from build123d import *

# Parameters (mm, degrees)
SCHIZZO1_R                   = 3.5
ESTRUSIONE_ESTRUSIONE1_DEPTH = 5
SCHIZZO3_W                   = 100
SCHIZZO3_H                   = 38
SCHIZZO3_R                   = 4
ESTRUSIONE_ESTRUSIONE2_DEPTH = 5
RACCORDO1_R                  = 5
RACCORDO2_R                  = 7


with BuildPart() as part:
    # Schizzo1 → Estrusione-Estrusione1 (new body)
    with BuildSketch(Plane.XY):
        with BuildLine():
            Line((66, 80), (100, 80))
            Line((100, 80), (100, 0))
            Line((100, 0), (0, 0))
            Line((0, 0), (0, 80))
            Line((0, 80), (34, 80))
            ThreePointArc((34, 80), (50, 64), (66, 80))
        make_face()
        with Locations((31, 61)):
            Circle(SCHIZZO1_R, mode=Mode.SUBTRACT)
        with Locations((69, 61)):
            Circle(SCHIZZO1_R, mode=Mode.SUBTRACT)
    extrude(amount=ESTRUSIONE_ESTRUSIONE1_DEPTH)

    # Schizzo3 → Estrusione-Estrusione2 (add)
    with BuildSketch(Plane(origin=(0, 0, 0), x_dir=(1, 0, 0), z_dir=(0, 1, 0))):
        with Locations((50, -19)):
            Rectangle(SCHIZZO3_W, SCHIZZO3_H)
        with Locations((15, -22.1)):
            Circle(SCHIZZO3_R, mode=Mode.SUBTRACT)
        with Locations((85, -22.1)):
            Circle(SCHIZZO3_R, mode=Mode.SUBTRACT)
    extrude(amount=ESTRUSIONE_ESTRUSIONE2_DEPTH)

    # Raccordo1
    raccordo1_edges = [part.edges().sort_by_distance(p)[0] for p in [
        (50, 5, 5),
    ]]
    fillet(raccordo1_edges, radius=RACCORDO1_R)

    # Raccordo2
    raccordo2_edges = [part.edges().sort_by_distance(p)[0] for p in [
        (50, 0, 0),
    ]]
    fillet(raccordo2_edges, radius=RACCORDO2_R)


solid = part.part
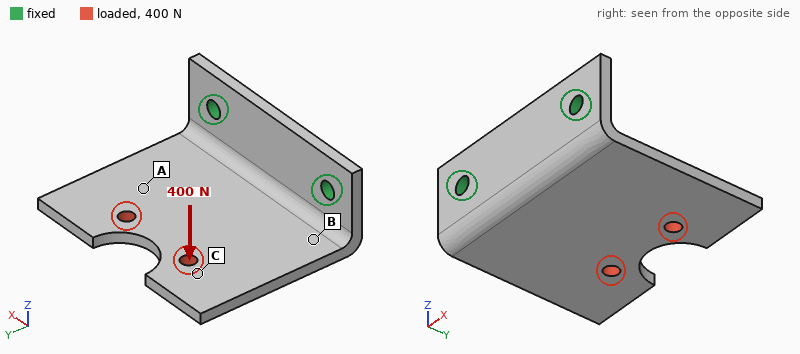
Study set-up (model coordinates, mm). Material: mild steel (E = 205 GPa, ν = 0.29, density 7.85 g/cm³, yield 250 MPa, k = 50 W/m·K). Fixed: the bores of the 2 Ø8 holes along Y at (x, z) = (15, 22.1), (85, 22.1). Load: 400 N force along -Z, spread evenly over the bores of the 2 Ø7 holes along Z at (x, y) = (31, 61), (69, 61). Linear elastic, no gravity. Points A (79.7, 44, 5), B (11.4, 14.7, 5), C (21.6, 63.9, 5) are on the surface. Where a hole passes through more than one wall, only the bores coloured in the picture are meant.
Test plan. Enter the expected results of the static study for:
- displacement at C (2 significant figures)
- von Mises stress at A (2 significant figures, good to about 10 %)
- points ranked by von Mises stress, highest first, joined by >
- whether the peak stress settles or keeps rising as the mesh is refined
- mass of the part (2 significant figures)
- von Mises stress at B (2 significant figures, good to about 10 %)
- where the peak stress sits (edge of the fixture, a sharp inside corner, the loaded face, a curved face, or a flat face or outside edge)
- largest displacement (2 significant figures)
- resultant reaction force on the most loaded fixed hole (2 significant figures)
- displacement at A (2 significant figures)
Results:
0.23 mm
17 MPa
B > A > C
keeps rising
420 g
38 MPa
edge of the fixture
0.31 mm
210 N
0.14 mm
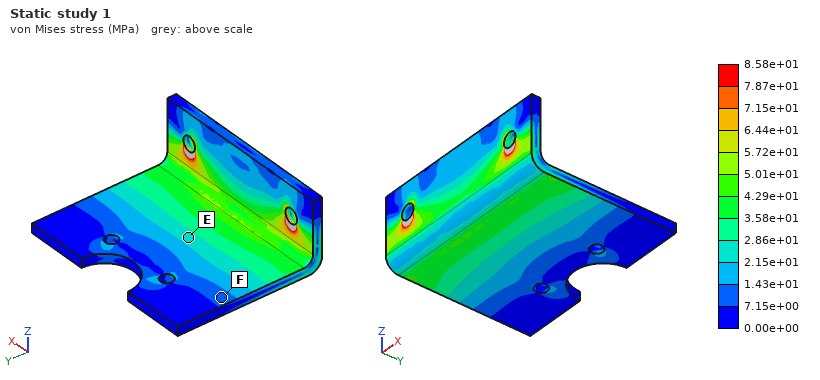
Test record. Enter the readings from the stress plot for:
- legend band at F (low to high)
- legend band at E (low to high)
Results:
7.15e+00 to 1.43e+01 MPa
2.15e+01 to 2.86e+01 MPa
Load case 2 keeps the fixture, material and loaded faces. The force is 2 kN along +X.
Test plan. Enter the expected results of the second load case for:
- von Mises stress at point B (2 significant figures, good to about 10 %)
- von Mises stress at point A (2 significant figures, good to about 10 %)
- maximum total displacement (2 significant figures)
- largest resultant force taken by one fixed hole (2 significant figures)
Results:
46 MPa
17 MPa
0.11 mm
1.9 kN
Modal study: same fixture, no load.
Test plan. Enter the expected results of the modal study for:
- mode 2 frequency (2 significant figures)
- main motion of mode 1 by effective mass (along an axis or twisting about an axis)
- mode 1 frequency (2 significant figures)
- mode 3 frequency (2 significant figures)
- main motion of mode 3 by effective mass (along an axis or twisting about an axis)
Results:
1200 Hz
along Z
570 Hz
2300 Hz
along X
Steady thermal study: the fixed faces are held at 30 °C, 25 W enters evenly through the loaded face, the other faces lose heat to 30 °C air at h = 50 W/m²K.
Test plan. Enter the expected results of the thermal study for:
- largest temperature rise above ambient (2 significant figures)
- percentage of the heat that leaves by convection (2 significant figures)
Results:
45 K
73 %
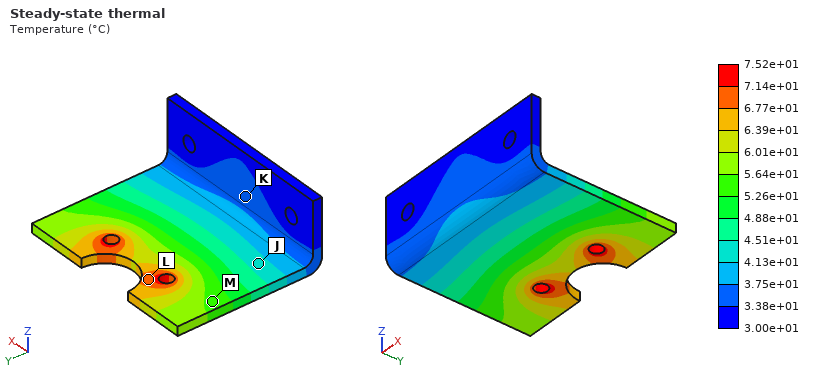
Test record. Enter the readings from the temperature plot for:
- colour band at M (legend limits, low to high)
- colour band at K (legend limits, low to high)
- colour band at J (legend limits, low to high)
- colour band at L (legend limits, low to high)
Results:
5.26e+01 to 5.64e+01 °C
3.38e+01 to 3.75e+01 °C
4.13e+01 to 4.51e+01 °C
6.77e+01 to 7.14e+01 °C
